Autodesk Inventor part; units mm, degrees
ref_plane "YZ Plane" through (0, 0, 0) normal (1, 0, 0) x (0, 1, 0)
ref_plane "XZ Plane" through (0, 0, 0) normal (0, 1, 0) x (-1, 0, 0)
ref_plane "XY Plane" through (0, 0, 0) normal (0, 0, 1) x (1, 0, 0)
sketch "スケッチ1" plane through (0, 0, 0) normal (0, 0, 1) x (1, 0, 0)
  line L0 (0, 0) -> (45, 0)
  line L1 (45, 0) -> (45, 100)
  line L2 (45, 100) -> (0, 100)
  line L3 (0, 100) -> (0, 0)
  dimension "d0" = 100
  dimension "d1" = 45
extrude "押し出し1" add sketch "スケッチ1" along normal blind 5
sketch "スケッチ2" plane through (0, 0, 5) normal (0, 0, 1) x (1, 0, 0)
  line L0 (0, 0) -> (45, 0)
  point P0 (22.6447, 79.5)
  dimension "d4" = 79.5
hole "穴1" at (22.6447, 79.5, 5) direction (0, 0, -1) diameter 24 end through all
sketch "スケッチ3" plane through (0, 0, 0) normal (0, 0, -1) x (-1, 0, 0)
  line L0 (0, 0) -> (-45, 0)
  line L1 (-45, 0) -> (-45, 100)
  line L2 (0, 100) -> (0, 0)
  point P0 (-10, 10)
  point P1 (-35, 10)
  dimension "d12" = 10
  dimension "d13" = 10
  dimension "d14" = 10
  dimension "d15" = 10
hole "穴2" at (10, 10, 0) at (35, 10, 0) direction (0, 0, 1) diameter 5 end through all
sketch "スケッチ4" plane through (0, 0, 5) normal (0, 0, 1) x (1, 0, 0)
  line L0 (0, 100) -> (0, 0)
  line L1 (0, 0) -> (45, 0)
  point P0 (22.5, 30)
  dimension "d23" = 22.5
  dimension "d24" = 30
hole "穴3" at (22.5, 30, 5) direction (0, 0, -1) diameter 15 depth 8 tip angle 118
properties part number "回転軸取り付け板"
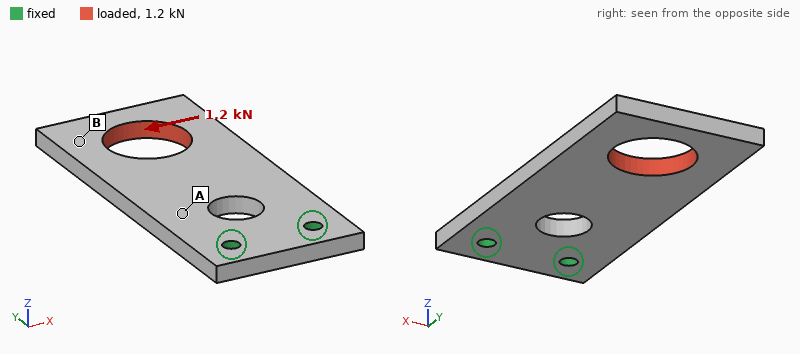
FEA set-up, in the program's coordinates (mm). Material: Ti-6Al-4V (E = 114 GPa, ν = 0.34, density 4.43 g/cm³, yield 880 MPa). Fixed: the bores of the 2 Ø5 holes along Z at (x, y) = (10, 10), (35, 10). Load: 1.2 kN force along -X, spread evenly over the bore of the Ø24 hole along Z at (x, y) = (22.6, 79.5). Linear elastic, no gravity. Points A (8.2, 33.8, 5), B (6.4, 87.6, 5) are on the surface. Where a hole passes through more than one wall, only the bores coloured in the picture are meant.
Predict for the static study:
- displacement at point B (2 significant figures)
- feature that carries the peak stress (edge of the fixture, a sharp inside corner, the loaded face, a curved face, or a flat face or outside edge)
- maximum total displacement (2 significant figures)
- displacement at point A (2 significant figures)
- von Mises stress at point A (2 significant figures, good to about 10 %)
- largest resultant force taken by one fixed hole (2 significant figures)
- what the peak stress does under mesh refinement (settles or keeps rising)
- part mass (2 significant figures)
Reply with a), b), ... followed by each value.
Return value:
a) 71 µm
b) edge of the fixture
c) 84 µm
d) 17 µm
e) 24 MPa
f) 3.0 kN
g) keeps rising
h) 85 g
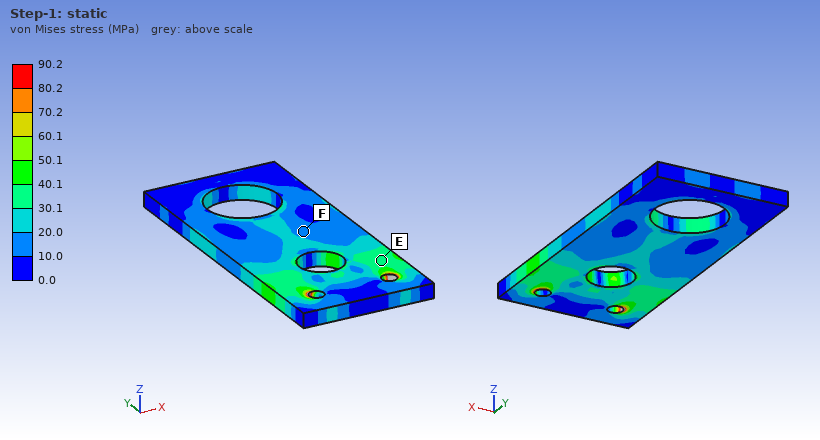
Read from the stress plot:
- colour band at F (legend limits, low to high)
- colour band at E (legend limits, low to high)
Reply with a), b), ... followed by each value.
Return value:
a) 10.0 to 20.0 MPa
b) 30.1 to 40.1 MPa
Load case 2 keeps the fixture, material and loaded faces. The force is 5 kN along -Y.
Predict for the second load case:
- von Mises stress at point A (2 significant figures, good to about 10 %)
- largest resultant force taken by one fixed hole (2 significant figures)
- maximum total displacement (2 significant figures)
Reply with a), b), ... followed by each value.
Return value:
a) 30 MPa
b) 2.5 kN
c) 30 µm
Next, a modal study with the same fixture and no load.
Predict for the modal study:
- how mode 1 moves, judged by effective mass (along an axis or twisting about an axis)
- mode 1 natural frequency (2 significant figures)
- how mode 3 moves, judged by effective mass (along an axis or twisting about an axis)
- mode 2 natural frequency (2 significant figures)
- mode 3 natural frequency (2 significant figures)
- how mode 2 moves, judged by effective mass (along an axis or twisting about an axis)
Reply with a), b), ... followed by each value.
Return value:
a) along Z
b) 530 Hz
c) along Z
d) 1900 Hz
e) 2900 Hz
f) twisting about Y
